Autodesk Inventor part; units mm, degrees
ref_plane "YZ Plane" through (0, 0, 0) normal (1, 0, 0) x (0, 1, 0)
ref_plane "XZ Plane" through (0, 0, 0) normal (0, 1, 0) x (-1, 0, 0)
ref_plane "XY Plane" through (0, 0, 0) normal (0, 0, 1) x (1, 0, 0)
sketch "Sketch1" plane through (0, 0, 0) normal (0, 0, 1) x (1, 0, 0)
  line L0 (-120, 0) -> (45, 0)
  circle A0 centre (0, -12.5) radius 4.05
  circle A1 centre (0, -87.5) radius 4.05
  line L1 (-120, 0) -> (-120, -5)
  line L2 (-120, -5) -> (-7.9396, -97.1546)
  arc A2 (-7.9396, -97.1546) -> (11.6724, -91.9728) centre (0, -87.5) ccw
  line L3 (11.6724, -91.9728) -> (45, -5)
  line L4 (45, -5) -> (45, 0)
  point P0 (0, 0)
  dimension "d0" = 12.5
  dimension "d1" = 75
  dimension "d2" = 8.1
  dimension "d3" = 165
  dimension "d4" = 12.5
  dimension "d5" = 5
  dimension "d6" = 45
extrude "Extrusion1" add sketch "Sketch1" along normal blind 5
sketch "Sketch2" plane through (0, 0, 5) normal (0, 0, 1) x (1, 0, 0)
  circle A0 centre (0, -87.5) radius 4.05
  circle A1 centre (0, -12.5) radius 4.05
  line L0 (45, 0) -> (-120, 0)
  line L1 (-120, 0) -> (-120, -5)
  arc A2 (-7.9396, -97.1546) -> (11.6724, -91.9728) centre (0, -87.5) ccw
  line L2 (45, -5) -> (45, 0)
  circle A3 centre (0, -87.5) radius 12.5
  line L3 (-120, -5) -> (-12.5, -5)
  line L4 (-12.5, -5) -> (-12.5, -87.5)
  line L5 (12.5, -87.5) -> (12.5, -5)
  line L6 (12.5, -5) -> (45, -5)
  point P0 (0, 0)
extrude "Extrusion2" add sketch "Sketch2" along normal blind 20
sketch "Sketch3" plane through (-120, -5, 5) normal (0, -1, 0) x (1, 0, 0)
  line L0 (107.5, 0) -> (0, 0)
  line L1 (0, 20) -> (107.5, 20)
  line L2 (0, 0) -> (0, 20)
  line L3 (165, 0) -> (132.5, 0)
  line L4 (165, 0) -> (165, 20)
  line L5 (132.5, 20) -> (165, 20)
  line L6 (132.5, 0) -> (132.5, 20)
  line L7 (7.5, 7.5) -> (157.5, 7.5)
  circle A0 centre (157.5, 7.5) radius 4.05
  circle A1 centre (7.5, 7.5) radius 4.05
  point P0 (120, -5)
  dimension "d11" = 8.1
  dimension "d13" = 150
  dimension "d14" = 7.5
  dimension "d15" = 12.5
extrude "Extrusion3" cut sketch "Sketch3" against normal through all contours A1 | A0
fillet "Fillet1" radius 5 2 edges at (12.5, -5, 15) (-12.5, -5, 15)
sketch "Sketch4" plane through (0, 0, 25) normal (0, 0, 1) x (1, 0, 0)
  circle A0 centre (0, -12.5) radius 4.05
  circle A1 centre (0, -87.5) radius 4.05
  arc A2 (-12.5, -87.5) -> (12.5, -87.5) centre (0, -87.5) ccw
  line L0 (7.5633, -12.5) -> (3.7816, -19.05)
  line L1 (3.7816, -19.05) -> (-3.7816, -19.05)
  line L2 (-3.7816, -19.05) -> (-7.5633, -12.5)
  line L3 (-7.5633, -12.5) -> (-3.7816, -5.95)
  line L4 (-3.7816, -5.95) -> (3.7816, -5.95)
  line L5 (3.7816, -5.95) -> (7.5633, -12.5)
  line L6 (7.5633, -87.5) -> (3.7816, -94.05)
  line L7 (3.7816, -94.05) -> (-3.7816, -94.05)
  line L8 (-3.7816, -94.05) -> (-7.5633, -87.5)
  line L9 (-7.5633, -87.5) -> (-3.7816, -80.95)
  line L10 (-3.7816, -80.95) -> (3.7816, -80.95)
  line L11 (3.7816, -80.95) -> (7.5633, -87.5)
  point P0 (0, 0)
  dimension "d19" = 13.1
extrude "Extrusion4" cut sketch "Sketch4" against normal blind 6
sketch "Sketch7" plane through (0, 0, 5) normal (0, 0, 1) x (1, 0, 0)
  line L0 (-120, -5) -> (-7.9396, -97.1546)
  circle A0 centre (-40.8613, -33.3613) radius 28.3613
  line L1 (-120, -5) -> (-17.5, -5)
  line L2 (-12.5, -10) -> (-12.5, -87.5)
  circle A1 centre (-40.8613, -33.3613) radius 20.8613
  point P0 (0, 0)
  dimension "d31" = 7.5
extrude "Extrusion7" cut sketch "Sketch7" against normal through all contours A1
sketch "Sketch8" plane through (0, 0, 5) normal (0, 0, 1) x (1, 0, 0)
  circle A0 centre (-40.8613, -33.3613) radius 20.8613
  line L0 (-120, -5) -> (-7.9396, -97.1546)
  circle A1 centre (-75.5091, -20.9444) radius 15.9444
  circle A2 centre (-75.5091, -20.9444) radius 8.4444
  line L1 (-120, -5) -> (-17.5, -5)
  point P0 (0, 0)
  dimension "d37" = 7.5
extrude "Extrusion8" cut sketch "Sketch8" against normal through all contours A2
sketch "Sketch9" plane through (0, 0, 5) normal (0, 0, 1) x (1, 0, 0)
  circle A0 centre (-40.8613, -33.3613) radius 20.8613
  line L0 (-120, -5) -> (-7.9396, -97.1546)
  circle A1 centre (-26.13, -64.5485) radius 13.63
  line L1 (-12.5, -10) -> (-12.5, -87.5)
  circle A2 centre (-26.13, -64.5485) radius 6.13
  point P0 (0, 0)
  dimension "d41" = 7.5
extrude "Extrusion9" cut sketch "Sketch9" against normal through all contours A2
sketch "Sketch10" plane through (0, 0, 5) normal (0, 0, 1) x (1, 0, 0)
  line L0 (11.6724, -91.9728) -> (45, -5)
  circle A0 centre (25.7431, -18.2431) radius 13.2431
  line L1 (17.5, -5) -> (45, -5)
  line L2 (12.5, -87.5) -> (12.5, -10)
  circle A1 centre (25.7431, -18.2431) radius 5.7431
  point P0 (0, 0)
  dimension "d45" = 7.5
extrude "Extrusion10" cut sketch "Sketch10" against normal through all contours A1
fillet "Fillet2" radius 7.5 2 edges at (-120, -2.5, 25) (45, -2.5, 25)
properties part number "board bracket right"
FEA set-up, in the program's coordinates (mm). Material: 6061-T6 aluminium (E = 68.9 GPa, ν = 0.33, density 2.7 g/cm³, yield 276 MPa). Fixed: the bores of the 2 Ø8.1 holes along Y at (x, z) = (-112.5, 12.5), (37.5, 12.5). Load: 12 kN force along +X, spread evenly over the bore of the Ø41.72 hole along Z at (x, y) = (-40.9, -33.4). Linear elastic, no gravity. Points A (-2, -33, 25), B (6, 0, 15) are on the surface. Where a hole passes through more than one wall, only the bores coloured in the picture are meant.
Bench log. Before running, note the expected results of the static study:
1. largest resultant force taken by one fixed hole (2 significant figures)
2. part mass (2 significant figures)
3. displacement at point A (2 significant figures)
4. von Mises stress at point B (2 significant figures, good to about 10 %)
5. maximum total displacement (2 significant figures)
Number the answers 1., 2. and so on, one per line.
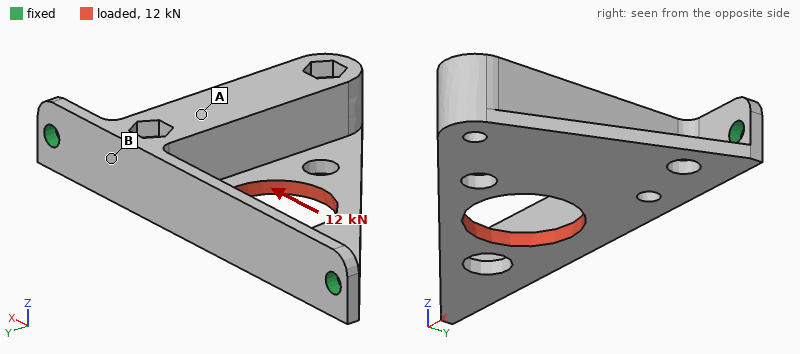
1. 6.5 kN
2. 260 g
3. 0.094 mm
4. 26 MPa
5. 0.23 mm
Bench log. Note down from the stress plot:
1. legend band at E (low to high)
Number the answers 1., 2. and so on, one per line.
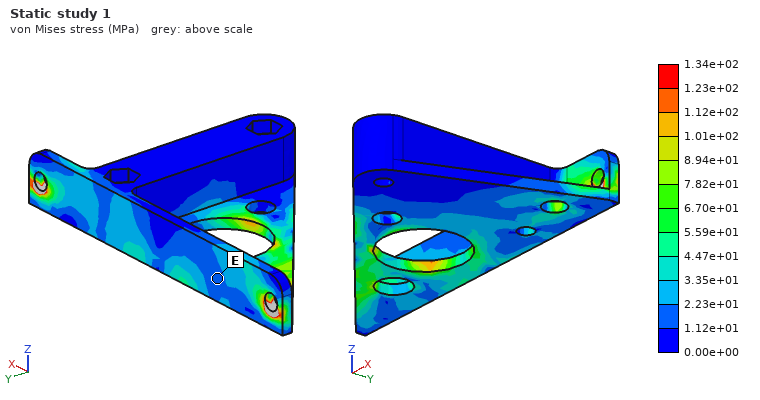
1. 1.12e+01 to 2.23e+01 MPa
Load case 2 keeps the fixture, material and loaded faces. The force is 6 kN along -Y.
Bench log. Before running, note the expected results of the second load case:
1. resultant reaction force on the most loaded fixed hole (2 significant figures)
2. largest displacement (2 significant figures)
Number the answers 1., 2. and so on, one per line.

1. 3.8 kN
2. 0.51 mm
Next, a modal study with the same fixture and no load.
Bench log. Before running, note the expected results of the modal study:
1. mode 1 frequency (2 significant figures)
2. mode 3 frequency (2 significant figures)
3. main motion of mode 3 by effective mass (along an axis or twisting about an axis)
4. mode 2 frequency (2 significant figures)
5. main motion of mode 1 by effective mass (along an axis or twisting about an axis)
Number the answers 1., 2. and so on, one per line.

1. 390 Hz
2. 2700 Hz
3. along Y
4. 2100 Hz
5. along Z
